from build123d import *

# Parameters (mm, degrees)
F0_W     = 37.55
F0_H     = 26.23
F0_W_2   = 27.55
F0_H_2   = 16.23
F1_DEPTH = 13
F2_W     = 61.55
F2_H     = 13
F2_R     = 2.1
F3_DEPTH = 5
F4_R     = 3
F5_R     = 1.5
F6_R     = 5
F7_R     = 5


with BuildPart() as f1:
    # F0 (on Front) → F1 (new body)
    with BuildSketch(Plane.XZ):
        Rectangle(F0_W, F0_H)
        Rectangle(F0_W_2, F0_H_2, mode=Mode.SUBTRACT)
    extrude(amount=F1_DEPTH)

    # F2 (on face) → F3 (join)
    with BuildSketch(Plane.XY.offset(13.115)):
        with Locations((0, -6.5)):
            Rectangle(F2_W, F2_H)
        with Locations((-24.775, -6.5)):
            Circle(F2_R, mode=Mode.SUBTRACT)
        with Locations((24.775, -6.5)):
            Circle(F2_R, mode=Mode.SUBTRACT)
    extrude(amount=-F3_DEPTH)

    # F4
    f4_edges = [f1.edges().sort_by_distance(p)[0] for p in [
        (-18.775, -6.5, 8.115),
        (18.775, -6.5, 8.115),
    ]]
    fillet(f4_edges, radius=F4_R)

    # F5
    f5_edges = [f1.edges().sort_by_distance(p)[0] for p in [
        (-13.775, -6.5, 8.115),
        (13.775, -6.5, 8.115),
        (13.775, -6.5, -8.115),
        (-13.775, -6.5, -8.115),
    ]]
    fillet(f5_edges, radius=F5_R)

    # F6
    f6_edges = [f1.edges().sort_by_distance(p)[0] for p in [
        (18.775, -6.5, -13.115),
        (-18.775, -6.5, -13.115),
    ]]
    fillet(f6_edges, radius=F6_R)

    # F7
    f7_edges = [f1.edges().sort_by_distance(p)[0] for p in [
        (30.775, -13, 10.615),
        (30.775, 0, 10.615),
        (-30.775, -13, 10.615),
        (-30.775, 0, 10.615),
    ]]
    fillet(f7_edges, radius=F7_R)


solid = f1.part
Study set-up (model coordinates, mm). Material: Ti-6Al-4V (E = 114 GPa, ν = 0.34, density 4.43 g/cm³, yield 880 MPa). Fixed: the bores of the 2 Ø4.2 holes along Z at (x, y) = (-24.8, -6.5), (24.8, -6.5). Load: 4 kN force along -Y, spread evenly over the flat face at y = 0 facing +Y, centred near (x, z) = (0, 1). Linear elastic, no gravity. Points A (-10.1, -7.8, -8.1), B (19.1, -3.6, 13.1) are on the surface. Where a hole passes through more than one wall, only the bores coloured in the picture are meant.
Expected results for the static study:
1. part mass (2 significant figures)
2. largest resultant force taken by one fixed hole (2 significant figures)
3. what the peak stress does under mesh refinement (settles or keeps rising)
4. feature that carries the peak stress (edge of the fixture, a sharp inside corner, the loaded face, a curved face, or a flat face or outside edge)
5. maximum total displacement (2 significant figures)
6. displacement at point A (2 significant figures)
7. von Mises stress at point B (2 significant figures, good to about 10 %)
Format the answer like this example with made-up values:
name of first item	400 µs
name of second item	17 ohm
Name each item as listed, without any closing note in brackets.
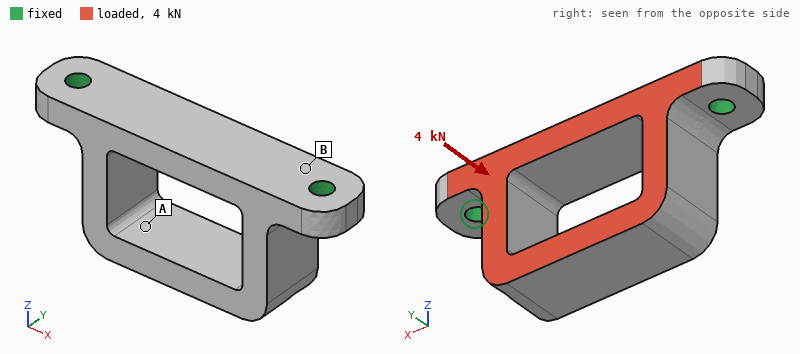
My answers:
part mass	37 g
largest resultant force taken by one fixed hole	2.0 kN
what the peak stress does under mesh refinement	keeps rising
feature that carries the peak stress	edge of the fixture
maximum total displacement	0.15 mm
displacement at point A	0.12 mm
von Mises stress at point B	100 MPa
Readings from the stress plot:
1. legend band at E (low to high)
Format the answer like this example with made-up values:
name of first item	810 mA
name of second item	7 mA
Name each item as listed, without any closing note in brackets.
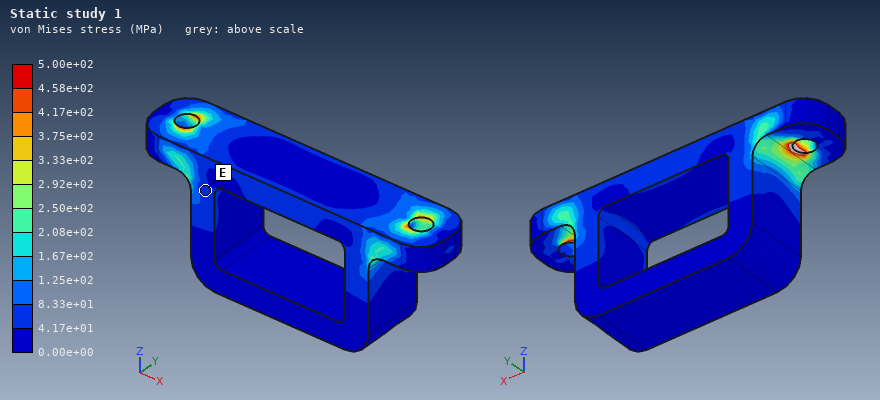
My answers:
legend band at E	4.17e+01 to 8.33e+01 MPa
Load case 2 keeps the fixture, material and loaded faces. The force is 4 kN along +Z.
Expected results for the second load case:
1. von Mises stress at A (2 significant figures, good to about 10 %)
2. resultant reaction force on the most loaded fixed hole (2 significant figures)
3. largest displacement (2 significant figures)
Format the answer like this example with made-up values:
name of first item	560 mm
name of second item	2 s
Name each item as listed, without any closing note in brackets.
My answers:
von Mises stress at A	35 MPa
resultant reaction force on the most loaded fixed hole	2.0 kN
largest displacement	0.11 mm
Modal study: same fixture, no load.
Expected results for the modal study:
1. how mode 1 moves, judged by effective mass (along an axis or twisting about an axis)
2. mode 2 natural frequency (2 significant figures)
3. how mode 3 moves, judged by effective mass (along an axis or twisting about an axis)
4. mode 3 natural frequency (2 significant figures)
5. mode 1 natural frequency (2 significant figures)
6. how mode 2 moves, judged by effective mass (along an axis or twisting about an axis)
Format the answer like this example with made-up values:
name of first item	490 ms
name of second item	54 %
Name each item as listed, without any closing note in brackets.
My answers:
how mode 1 moves, judged by effective mass	along Y
mode 2 natural frequency	7600 Hz
how mode 3 moves, judged by effective mass	twisting about Z
mode 3 natural frequency	10 kHz
mode 1 natural frequency	5000 Hz
how mode 2 moves, judged by effective mass	along X
